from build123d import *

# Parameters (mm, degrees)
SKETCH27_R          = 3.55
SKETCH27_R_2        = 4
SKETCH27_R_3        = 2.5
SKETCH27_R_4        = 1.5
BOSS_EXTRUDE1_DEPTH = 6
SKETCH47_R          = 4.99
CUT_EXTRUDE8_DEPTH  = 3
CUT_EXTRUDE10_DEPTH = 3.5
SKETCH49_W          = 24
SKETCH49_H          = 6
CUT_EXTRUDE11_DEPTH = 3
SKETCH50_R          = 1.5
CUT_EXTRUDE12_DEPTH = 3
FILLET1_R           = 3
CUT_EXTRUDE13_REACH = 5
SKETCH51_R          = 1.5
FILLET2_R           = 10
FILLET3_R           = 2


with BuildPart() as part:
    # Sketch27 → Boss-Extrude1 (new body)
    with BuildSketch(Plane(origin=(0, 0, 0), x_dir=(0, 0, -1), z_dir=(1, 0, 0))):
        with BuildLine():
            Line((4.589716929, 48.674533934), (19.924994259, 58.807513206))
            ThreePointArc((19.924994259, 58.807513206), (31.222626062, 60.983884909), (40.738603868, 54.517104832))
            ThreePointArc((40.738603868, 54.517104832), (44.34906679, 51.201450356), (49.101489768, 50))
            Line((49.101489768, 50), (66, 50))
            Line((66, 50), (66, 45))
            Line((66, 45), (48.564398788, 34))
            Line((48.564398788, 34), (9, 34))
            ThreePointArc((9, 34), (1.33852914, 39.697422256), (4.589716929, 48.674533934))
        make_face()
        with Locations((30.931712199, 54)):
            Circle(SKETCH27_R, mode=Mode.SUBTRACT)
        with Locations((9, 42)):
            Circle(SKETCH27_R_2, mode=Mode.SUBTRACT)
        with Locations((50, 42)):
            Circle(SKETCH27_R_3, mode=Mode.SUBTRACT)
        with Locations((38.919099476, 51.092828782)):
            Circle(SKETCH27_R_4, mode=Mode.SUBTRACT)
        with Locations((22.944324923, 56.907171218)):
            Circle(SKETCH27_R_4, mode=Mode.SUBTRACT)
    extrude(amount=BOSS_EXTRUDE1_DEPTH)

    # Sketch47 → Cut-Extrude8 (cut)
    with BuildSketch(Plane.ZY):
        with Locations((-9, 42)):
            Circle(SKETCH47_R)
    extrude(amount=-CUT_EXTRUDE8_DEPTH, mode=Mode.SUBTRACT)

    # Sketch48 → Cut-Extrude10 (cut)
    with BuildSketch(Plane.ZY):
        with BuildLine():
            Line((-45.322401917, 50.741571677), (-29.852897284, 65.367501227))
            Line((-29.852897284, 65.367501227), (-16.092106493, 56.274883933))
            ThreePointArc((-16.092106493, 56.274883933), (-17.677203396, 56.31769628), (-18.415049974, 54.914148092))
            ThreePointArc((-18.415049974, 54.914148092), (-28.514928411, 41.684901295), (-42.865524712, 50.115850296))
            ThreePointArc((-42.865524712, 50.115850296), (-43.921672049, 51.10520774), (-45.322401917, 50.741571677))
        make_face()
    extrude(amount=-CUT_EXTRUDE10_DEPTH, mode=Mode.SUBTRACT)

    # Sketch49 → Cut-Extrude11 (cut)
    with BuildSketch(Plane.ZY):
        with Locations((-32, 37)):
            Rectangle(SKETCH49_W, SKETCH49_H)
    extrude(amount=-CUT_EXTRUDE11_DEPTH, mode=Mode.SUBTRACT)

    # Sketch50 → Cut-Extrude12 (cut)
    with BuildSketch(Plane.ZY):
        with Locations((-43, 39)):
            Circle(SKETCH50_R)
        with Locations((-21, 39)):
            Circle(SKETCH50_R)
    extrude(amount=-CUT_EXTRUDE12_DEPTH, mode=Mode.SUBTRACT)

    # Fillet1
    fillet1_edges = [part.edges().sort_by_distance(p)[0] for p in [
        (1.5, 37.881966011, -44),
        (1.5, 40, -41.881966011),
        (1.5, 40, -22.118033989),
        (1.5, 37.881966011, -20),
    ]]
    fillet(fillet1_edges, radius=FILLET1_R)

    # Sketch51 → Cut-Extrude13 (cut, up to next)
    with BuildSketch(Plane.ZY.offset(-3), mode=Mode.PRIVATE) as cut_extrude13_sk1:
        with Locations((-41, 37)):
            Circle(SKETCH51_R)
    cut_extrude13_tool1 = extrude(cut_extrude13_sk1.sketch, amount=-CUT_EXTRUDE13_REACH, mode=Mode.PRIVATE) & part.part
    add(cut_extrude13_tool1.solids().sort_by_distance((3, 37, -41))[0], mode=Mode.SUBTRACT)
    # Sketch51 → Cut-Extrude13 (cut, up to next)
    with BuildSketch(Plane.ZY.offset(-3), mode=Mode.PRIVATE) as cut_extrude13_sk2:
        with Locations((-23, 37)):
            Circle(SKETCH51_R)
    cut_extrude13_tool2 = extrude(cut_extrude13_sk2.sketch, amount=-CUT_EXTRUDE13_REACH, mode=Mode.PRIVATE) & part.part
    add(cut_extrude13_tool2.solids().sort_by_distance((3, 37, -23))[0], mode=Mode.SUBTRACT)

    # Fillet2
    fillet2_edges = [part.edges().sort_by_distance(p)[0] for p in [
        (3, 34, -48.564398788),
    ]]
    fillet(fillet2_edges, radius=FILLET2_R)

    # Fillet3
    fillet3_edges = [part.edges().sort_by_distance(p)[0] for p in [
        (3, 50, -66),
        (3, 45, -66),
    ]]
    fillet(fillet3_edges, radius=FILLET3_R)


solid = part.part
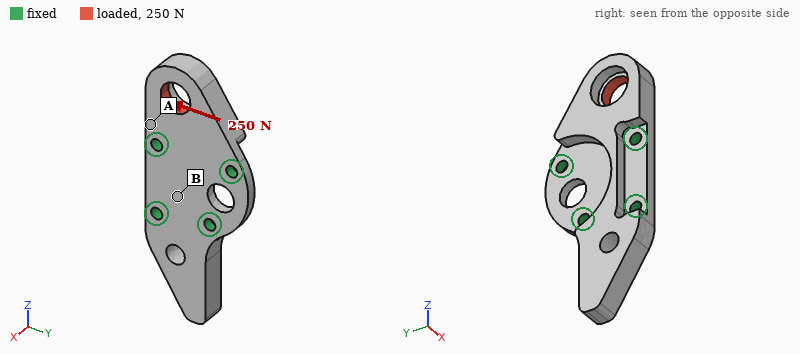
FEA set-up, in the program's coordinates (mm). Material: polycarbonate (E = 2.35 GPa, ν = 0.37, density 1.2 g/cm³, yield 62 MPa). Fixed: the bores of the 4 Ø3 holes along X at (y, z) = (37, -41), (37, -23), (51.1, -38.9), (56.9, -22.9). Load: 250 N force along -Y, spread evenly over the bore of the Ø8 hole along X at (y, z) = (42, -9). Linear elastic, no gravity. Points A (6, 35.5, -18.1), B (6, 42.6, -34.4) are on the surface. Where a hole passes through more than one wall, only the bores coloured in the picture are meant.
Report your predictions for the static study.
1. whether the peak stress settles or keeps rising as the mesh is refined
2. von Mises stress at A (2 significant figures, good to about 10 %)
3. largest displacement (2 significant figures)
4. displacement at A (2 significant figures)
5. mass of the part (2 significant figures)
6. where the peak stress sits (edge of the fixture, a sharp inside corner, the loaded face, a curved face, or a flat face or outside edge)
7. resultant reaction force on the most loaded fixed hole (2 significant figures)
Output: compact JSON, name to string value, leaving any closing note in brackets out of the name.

{"whether the peak stress settles or keeps rising as the mesh is refined": "keeps rising", "von Mises stress at A": "8.3 MPa", "largest displacement": "0.20 mm", "displacement at A": "0.038 mm", "mass of the part": "5.6 g", "where the peak stress sits": "edge of the fixture", "resultant reaction force on the most loaded fixed hole": "210 N"}
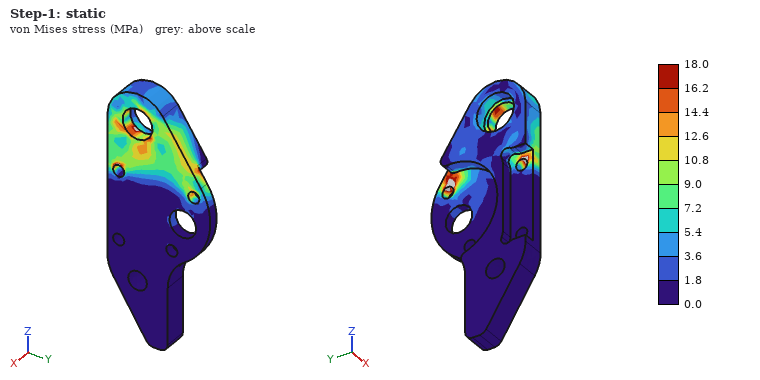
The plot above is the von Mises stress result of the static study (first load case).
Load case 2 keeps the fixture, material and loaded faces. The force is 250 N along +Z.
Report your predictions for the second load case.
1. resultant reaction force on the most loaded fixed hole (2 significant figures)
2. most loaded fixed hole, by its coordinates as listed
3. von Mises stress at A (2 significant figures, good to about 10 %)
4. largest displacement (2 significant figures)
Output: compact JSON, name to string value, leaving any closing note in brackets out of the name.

{"resultant reaction force on the most loaded fixed hole": "160 N", "most loaded fixed hole, by its coordinates as listed": "(37, -23)", "von Mises stress at A": "8.3 MPa", "largest displacement": "0.11 mm"}
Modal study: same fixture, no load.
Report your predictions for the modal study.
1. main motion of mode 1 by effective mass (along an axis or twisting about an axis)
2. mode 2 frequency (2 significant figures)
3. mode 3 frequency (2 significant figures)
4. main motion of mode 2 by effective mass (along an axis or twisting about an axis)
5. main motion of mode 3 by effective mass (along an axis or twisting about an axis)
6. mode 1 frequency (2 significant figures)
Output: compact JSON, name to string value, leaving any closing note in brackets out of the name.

{"main motion of mode 1 by effective mass": "along X", "mode 2 frequency": "2000 Hz", "mode 3 frequency": "4900 Hz", "main motion of mode 2 by effective mass": "along X", "main motion of mode 3 by effective mass": "along Y", "mode 1 frequency": "1700 Hz"}
